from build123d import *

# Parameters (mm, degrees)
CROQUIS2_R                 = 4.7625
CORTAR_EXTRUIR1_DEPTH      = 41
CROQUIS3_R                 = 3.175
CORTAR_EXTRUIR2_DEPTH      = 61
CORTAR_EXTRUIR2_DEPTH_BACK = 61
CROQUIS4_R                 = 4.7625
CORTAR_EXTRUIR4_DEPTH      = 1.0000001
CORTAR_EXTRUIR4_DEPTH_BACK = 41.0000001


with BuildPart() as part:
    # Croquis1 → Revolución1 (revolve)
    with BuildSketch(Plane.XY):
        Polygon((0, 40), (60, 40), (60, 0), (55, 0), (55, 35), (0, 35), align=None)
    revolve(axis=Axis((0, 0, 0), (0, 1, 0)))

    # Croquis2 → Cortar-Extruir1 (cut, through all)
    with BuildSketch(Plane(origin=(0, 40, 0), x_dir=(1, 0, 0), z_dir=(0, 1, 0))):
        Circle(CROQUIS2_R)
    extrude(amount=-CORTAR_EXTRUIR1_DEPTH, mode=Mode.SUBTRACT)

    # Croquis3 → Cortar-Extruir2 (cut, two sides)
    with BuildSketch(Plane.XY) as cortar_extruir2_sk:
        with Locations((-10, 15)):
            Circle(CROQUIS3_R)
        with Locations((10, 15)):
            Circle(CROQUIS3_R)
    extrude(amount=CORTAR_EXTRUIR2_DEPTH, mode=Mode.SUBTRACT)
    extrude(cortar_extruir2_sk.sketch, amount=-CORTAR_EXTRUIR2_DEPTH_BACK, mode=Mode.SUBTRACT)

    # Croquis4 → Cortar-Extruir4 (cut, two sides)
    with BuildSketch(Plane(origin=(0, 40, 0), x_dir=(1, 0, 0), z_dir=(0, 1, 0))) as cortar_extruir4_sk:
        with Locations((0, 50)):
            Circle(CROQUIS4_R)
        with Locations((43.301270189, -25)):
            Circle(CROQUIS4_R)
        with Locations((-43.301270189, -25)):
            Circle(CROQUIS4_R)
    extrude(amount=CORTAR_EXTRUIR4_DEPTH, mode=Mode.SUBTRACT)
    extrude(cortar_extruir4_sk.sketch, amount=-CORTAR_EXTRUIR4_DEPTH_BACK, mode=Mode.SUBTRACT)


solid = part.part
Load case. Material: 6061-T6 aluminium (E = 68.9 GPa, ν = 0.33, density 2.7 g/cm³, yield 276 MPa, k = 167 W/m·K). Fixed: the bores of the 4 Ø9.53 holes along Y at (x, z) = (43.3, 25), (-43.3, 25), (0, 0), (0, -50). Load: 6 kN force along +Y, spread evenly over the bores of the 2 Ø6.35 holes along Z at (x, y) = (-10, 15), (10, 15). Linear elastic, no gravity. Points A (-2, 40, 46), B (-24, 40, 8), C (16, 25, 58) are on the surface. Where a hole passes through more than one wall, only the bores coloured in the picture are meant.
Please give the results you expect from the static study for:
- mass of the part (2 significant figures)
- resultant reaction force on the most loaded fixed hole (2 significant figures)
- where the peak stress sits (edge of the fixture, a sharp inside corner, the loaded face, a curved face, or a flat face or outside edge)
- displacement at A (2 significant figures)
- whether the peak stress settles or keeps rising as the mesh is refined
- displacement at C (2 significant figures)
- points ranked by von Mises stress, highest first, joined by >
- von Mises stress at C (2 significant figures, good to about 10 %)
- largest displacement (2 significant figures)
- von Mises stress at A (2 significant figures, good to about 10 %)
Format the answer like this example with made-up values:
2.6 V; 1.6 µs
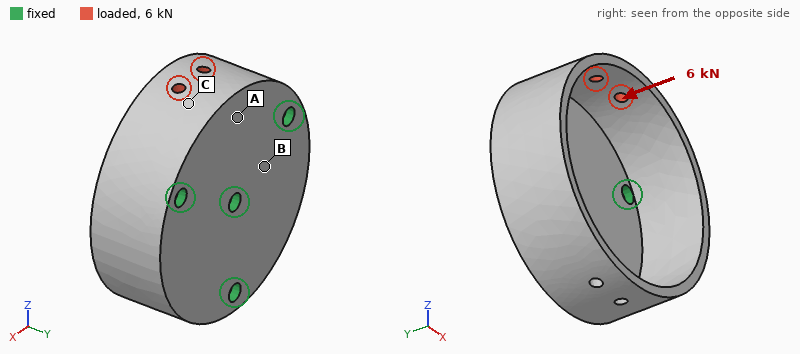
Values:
320 g; 3.6 kN; edge of the fixture; 0.19 mm; keeps rising; 0.32 mm; C > A > B; 78 MPa; 0.58 mm; 39 MPa
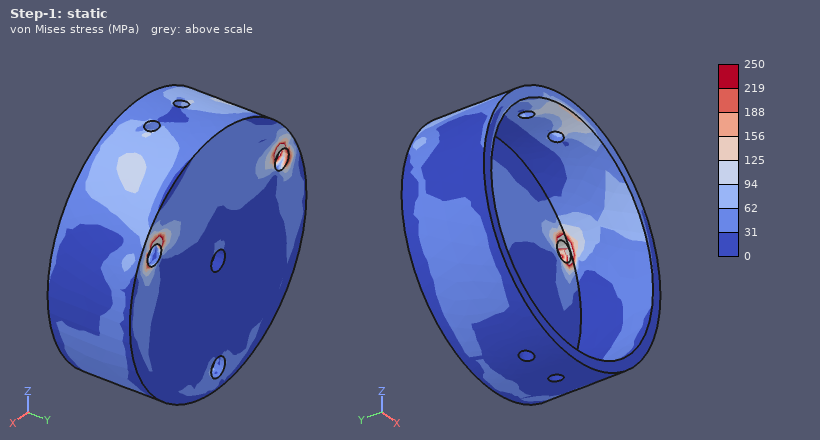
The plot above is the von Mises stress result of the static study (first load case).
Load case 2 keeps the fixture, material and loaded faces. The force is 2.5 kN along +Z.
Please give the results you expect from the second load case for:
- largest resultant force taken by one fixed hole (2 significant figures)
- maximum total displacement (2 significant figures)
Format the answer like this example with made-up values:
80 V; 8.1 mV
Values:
1.6 kN; 0.27 mm
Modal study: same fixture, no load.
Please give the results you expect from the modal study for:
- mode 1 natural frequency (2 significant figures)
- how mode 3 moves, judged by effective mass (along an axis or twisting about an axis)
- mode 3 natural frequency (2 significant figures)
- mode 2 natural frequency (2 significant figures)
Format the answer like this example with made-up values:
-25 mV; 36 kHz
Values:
2200 Hz; along Y; 4000 Hz; 2200 Hz
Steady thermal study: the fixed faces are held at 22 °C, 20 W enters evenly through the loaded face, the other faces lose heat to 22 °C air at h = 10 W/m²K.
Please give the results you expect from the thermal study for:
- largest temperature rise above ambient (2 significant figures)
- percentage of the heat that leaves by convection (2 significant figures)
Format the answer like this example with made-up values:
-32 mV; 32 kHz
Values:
14 K; 5.4 %
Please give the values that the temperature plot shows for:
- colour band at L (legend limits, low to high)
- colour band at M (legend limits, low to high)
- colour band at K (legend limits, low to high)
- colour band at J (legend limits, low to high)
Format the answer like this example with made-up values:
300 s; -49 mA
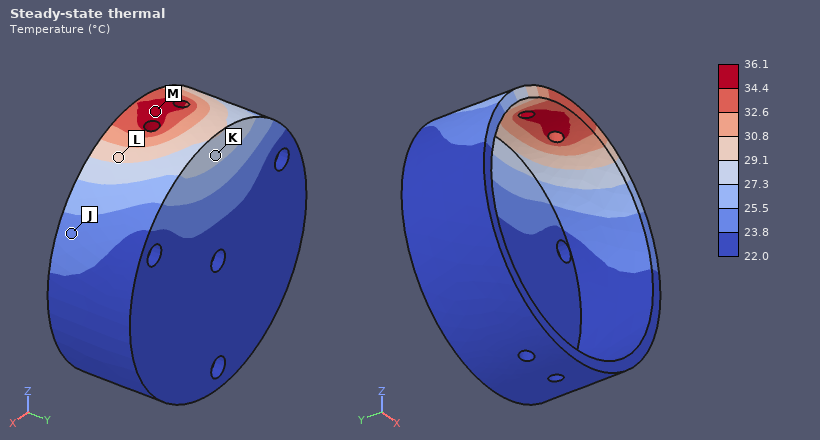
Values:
29.1 to 30.8 °C; 34.4 to 36.1 °C; 27.3 to 29.1 °C; 23.8 to 25.5 °C
